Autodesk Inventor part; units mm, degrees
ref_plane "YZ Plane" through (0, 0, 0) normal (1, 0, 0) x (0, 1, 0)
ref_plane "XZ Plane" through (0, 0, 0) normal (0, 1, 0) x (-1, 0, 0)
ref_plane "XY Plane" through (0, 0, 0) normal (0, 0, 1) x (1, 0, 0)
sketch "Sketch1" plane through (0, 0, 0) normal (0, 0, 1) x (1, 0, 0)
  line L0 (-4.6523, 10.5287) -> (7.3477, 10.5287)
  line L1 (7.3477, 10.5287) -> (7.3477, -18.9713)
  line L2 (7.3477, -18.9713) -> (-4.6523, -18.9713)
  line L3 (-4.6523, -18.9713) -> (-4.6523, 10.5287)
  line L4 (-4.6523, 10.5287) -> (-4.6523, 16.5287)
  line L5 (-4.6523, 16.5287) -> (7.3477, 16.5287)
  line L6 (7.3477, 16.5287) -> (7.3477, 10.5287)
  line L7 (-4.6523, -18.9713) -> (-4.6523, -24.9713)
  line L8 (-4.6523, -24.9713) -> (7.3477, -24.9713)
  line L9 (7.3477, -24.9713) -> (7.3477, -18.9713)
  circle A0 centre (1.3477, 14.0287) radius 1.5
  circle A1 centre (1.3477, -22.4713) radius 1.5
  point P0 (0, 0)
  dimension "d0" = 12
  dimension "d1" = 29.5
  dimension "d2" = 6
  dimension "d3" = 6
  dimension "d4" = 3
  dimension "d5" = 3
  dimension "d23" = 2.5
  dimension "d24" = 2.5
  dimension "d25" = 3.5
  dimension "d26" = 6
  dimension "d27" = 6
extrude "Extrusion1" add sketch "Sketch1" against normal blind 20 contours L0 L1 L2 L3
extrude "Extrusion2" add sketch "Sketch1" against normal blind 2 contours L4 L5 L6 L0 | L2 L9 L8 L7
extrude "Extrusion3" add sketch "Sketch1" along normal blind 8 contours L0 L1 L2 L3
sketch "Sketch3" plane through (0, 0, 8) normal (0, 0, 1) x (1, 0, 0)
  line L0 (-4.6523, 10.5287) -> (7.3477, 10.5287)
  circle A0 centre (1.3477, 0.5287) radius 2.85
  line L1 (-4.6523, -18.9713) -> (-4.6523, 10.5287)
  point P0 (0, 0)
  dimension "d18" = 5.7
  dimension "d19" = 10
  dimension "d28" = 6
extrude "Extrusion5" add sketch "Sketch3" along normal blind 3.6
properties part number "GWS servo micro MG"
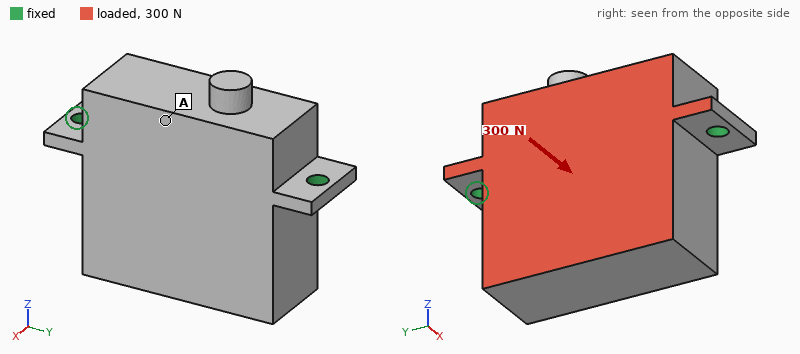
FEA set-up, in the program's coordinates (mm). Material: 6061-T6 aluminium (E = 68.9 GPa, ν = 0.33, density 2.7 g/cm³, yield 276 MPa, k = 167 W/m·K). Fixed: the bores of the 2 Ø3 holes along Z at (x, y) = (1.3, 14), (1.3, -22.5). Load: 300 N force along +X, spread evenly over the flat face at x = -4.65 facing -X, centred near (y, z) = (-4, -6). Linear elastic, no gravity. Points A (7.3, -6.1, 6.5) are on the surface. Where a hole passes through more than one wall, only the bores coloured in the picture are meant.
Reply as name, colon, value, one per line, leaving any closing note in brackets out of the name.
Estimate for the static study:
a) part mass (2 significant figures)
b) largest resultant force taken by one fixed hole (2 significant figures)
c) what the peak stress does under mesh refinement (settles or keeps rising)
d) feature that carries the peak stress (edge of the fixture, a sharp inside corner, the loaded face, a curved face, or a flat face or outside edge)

part mass: 28 g
largest resultant force taken by one fixed hole: 150 N
what the peak stress does under mesh refinement: keeps rising
feature that carries the peak stress: edge of the fixture
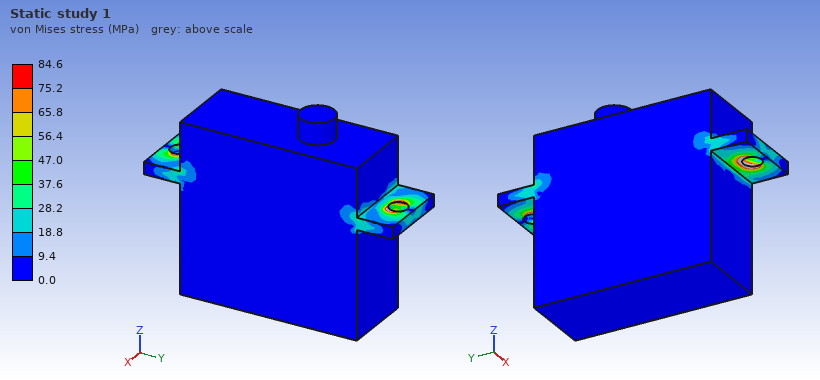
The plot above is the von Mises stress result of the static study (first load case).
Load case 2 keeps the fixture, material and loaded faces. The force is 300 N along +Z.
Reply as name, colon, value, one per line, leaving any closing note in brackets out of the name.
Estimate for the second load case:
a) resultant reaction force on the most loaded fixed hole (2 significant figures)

resultant reaction force on the most loaded fixed hole: 150 N
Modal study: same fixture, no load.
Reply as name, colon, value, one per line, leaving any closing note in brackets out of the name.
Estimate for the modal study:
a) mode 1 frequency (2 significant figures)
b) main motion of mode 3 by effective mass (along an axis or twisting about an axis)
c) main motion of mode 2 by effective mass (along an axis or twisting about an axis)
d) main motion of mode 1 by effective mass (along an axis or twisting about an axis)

mode 1 frequency: 2500 Hz
main motion of mode 3 by effective mass: along Y
main motion of mode 2 by effective mass: along Z
main motion of mode 1 by effective mass: along X
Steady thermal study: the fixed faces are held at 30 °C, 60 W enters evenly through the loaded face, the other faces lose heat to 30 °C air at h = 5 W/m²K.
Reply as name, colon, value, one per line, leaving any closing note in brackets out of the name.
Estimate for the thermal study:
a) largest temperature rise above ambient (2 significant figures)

largest temperature rise above ambient: 46 K
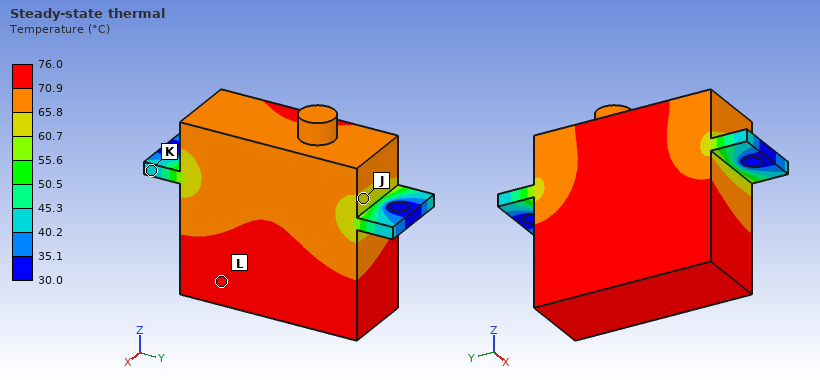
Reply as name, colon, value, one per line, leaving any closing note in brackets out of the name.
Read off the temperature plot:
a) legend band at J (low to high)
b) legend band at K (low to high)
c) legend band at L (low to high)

legend band at J: 60.7 to 65.8 °C
legend band at K: 40.2 to 45.3 °C
legend band at L: 70.9 to 76.0 °C
